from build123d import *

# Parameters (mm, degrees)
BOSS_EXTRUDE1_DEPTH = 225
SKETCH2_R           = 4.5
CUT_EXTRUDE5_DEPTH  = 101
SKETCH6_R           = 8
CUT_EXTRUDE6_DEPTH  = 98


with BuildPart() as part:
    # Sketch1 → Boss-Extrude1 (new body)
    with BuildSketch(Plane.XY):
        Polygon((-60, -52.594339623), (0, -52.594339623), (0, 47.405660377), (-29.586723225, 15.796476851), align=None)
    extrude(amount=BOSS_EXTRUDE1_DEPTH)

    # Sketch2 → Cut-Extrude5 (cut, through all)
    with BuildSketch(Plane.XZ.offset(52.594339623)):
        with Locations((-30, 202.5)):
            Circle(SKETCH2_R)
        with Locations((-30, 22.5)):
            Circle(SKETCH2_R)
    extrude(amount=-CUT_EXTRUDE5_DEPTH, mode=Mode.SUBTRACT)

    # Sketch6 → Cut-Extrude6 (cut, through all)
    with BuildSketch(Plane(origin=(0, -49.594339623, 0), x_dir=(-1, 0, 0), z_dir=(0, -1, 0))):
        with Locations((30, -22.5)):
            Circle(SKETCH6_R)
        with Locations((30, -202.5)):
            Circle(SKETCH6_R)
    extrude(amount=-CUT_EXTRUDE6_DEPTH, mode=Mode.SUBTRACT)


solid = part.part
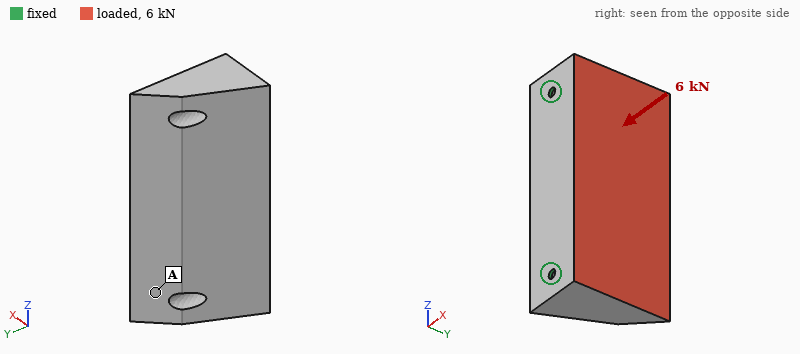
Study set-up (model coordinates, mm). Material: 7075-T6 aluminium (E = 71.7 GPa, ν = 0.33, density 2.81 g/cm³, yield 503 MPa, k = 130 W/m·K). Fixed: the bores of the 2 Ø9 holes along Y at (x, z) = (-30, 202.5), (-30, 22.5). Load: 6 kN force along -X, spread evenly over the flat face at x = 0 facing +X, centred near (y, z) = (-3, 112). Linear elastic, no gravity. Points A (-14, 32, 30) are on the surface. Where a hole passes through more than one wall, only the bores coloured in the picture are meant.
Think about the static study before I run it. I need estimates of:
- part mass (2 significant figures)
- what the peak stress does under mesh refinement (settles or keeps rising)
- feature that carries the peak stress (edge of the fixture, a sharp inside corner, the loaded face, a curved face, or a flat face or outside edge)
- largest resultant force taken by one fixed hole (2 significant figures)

2.2 kg
keeps rising
edge of the fixture
3.0 kN
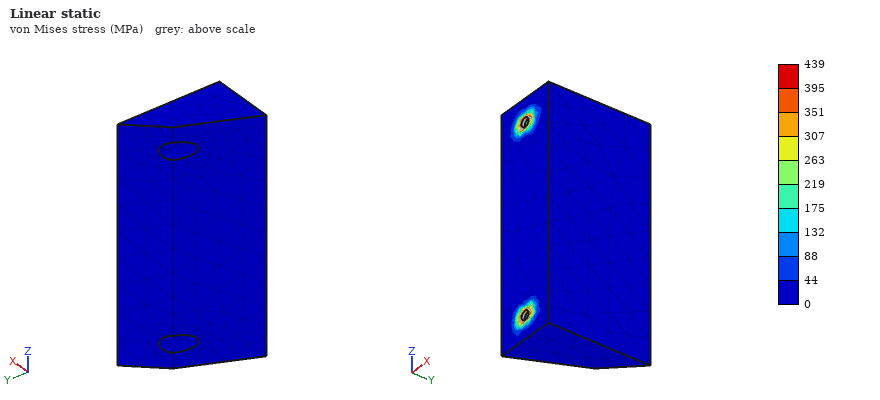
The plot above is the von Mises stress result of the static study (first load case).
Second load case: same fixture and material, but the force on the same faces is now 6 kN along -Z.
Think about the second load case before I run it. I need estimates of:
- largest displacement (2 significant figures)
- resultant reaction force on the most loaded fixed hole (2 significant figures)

18 µm
3.6 kN
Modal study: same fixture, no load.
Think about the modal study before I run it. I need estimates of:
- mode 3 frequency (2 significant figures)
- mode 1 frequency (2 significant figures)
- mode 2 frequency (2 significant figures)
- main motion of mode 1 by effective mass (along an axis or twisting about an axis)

2600 Hz
300 Hz
2500 Hz
along X
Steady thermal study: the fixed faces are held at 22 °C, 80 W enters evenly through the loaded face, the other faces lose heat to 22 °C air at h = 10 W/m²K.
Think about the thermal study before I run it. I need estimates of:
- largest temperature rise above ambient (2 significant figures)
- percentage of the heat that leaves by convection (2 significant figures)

21 K
11 %
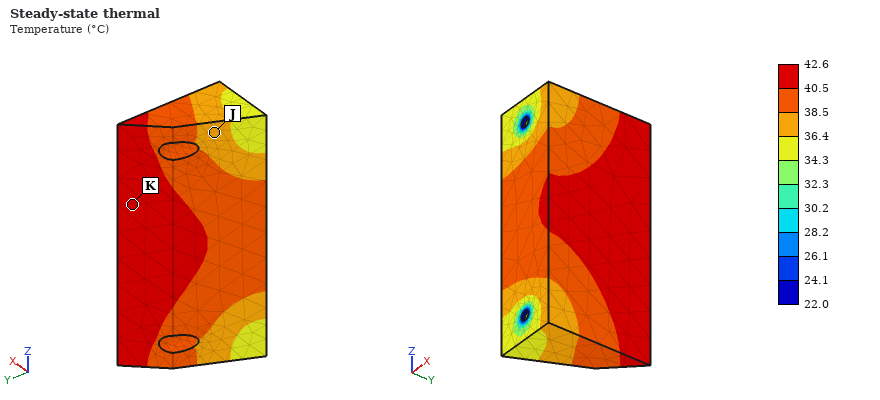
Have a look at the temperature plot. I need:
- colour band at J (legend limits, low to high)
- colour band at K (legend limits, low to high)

36.4 to 38.5 °C
40.5 to 42.6 °C
